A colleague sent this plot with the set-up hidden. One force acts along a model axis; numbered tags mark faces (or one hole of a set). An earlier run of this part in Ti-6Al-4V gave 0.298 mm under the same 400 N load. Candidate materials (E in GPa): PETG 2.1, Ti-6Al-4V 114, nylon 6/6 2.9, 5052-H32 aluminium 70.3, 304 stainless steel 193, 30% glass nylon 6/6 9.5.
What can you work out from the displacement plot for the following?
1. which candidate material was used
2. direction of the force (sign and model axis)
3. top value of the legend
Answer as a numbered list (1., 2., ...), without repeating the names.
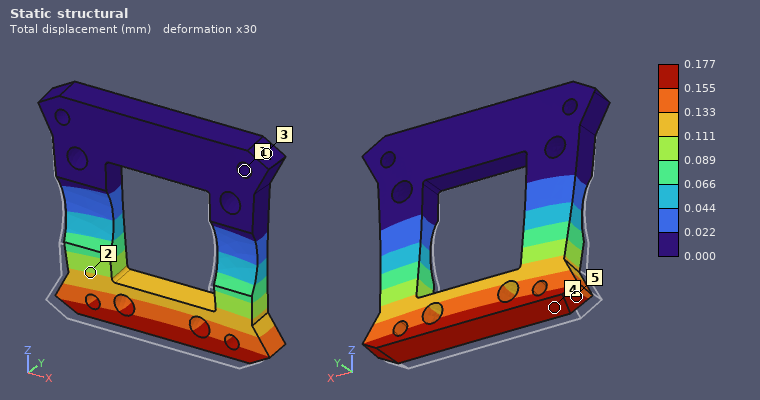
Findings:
1. 304 stainless steel
2. +Y
3. 0.177 mm
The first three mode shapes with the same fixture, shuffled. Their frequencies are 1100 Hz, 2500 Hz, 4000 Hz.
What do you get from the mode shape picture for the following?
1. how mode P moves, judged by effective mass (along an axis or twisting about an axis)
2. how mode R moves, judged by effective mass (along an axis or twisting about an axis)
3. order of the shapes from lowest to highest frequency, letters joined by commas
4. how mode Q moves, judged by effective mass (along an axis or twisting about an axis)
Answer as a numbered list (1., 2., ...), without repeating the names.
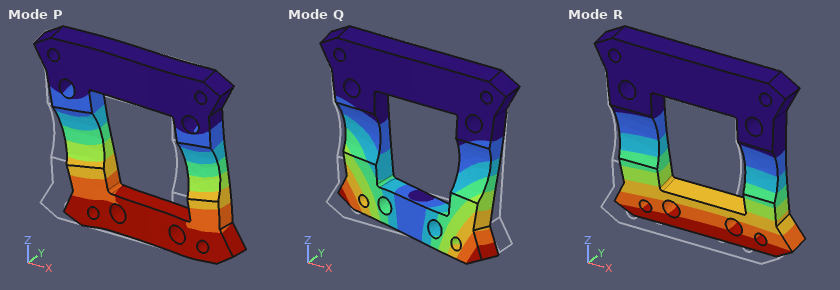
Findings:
1. along X
2. along Y
3. R, Q, P
4. twisting about Z
